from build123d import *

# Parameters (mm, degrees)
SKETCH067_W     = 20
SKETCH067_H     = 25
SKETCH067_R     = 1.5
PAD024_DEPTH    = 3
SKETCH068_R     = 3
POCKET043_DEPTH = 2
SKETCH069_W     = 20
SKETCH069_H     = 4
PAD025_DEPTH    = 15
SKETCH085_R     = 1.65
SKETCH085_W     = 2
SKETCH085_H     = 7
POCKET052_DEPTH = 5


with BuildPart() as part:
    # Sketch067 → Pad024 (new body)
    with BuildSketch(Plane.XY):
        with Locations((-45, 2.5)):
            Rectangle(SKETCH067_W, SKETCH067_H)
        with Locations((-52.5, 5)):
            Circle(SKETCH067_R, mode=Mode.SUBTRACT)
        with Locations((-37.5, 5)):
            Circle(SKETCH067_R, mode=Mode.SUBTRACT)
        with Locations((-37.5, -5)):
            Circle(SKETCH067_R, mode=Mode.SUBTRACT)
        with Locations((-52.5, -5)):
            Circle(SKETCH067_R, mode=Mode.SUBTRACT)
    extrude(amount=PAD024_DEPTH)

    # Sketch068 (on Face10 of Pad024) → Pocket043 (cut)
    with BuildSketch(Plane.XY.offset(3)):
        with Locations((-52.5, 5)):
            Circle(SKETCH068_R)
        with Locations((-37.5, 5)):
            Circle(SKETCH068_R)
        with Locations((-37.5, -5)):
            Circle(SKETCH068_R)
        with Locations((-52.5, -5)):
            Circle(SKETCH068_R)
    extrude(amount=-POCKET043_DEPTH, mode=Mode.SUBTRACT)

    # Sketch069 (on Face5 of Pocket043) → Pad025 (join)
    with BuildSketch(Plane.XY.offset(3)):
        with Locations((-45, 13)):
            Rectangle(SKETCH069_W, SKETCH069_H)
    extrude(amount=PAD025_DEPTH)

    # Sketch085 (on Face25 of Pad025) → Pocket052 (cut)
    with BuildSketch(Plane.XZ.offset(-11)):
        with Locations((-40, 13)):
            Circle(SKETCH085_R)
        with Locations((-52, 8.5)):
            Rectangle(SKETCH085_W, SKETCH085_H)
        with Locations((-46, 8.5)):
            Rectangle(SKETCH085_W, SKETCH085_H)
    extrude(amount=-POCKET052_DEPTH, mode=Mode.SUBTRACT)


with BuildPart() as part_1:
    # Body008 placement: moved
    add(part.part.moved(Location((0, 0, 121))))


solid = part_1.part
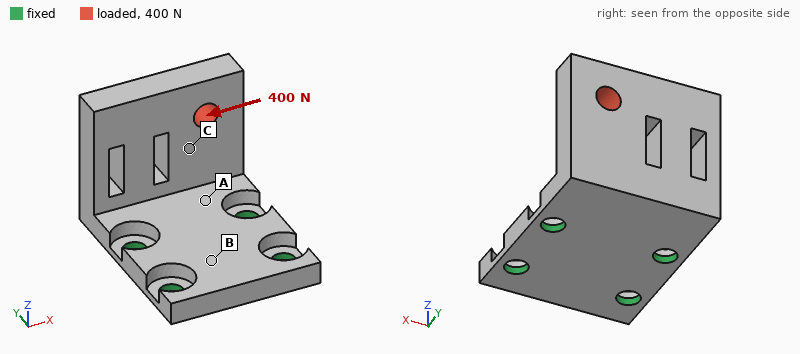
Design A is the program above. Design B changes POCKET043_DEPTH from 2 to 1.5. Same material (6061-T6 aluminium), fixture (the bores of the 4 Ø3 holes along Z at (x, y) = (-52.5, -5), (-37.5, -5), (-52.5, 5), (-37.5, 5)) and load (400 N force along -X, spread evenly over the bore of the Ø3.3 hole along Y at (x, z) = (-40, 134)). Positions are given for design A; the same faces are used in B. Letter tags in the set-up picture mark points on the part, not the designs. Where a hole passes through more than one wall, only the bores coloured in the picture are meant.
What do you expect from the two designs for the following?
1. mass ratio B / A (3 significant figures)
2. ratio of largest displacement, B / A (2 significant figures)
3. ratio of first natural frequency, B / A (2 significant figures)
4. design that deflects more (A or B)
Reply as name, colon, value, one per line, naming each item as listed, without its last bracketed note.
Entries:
mass ratio B / A: 1.02
ratio of largest displacement, B / A: 0.83
ratio of first natural frequency, B / A: 1.1
design that deflects more: A
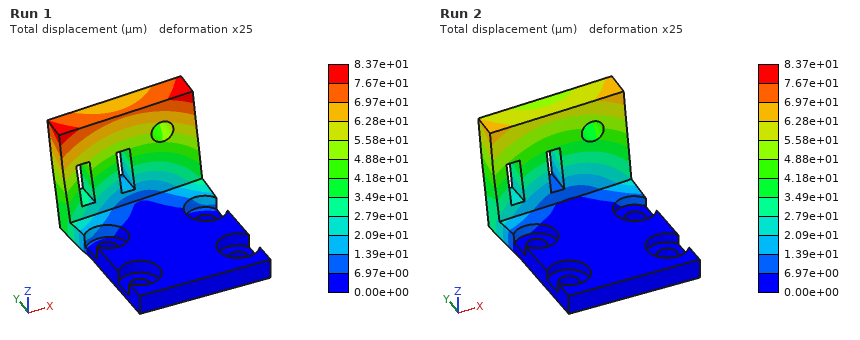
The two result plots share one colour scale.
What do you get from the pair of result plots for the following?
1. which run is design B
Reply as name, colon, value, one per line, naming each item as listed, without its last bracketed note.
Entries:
which run is design B: Run 2
